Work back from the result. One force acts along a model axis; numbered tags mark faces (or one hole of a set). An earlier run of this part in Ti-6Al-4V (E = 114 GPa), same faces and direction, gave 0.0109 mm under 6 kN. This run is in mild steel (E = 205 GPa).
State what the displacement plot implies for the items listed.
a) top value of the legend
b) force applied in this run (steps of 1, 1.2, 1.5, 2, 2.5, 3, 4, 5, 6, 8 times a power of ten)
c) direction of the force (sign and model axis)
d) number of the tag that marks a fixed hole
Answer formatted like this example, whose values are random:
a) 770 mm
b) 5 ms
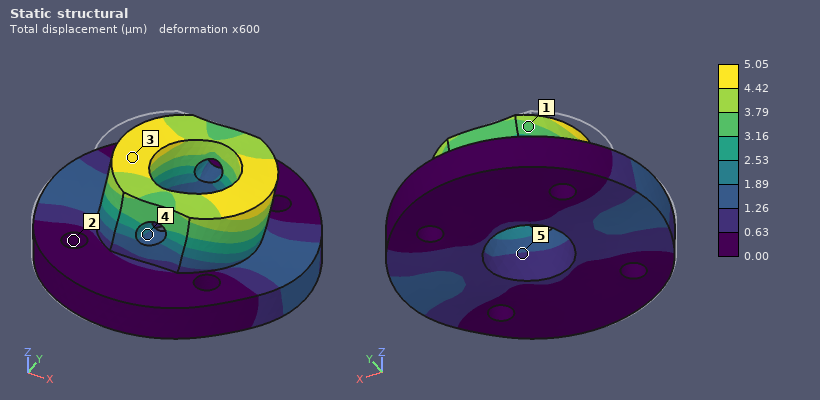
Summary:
a) 5.05 µm
b) 5 kN
c) +X
d) 2
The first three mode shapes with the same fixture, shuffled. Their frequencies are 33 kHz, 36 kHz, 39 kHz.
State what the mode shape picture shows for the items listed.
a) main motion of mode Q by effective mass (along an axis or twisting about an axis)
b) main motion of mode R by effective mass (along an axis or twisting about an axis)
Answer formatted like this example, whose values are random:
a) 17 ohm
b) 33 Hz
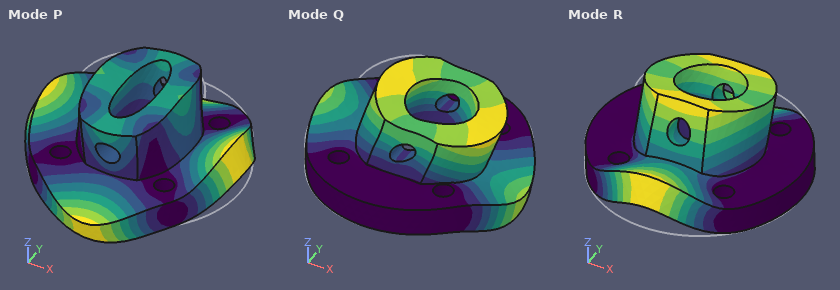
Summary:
a) along X
b) along Y
